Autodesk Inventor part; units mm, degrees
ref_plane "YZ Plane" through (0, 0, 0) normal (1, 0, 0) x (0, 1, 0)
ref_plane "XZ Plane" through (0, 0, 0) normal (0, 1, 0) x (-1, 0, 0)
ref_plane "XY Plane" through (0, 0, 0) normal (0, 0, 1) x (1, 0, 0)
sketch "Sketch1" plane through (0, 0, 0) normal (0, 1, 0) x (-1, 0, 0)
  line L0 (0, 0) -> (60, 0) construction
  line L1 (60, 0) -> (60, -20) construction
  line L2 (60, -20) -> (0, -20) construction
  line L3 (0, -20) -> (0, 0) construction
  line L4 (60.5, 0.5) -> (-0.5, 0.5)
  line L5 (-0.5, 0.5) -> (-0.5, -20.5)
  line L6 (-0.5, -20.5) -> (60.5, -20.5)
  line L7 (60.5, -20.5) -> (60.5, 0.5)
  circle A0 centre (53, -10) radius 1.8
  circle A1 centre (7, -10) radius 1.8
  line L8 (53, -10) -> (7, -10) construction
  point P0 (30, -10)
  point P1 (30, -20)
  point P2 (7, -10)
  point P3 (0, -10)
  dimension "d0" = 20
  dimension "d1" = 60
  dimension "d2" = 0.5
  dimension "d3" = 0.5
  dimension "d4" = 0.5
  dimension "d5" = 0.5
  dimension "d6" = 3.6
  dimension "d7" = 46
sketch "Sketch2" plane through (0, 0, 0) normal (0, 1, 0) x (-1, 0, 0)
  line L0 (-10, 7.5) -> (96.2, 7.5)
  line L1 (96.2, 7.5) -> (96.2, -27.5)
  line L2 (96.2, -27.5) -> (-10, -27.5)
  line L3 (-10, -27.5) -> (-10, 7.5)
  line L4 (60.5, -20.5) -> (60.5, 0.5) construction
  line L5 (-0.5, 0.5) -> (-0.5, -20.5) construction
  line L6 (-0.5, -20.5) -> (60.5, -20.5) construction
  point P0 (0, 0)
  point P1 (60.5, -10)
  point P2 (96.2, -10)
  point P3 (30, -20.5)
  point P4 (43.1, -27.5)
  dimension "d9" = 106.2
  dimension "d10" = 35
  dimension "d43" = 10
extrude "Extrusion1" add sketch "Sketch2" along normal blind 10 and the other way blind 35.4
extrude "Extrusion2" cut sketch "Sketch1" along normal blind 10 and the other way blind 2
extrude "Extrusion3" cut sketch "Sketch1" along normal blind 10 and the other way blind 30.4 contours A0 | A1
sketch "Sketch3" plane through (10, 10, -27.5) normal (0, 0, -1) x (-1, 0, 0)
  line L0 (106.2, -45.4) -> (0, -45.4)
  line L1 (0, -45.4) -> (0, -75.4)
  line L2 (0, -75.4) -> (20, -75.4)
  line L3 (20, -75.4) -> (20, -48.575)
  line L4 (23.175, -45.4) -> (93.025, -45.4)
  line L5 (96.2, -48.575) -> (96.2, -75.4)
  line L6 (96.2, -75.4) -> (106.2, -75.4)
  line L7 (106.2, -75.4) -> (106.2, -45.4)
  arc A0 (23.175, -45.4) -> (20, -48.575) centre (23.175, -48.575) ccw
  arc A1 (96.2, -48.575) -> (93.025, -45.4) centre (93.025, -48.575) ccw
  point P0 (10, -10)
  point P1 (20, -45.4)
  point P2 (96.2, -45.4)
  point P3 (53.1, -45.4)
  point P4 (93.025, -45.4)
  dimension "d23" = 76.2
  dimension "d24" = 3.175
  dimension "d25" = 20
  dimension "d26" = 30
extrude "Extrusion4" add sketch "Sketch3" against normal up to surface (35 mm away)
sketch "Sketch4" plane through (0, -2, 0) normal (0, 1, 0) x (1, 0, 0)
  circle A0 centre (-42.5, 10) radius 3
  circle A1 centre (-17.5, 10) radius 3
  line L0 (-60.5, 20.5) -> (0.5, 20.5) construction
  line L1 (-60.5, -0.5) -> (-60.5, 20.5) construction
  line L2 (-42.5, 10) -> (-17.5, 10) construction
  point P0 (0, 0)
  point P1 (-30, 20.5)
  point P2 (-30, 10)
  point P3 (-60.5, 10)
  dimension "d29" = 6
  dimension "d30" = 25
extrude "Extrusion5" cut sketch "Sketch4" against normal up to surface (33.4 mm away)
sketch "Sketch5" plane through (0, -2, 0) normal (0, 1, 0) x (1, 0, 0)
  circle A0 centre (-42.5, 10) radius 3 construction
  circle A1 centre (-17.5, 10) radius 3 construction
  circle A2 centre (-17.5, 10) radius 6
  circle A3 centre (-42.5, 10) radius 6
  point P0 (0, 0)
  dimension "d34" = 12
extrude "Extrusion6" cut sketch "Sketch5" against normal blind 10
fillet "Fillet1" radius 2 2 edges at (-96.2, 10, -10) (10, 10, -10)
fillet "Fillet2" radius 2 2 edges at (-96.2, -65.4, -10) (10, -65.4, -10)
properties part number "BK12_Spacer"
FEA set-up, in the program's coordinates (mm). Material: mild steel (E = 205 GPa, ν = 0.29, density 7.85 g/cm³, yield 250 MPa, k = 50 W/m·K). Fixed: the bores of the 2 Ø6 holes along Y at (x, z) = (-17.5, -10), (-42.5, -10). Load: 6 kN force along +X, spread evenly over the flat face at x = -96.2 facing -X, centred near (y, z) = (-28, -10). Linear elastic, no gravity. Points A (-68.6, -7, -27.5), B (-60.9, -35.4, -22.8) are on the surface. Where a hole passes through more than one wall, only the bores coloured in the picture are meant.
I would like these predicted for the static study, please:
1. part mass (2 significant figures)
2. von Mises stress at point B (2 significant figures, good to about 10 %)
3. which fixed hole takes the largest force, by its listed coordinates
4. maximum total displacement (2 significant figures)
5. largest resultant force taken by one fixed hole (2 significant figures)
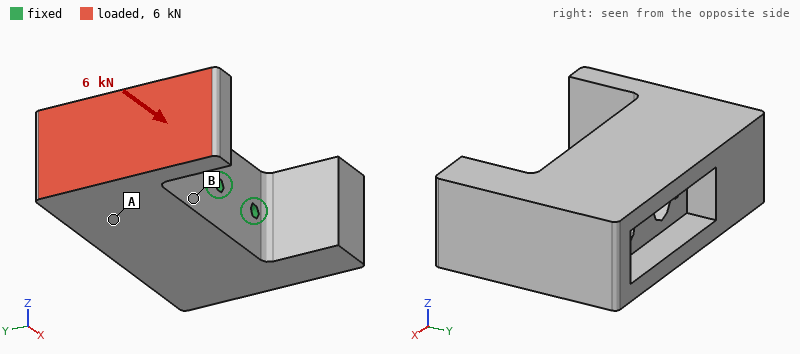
1.4 kg
11 MPa
(-42.5, -10)
28 µm
4.8 kN
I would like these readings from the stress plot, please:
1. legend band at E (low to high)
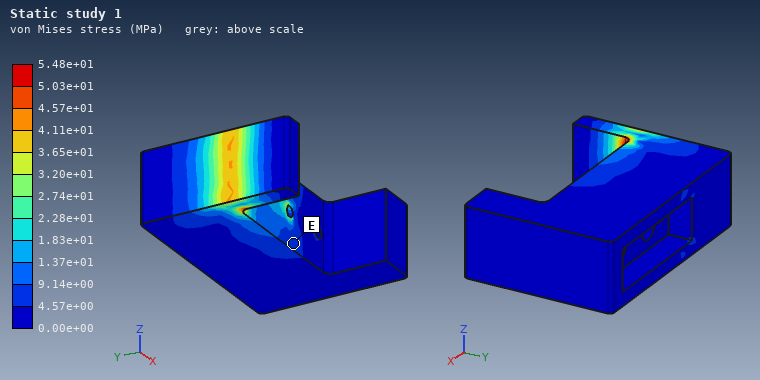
4.57e+00 to 9.14e+00 MPa
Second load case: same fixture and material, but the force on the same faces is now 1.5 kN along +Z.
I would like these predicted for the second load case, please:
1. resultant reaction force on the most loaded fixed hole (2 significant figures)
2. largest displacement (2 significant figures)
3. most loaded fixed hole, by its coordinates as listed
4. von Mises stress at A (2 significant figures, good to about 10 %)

4.0 kN
11 µm
(-42.5, -10)
4.9 MPa
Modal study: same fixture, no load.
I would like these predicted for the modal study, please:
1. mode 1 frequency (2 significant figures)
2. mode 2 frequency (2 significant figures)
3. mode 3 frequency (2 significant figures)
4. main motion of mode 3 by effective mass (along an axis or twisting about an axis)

4200 Hz
4300 Hz
5600 Hz
twisting about X
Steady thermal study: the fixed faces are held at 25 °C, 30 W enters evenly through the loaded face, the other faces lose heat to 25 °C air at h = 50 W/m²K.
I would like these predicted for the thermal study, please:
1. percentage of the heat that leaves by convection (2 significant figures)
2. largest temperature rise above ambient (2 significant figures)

29 %
30 K
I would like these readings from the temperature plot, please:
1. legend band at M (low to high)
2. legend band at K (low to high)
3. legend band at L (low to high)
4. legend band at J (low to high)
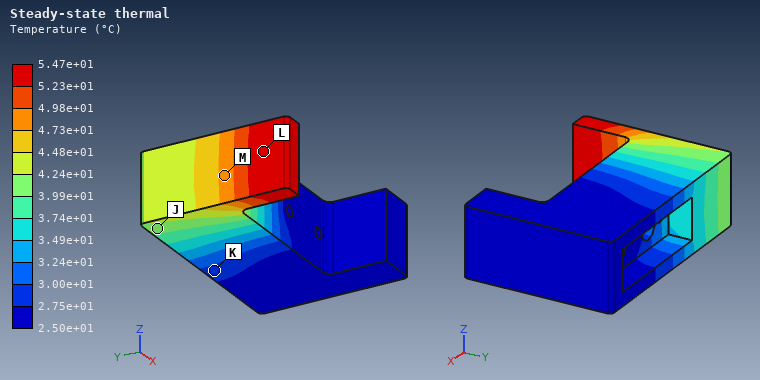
4.73e+01 to 4.98e+01 °C
2.75e+01 to 3.00e+01 °C
5.23e+01 to 5.47e+01 °C
3.99e+01 to 4.24e+01 °C
